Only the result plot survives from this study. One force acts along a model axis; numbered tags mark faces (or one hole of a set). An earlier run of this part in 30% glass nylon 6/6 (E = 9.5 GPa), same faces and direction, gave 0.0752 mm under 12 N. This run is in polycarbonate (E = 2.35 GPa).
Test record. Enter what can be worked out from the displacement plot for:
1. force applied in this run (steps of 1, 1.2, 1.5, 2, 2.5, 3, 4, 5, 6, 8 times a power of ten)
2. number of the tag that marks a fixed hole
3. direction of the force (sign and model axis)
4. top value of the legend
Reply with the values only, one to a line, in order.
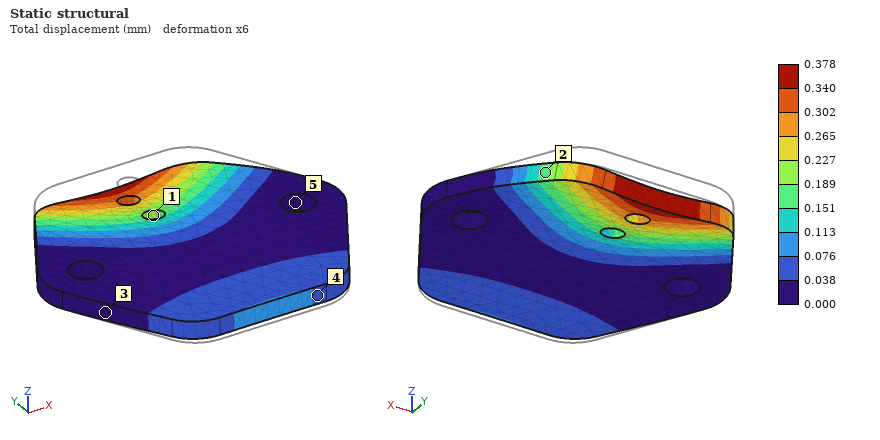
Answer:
15 N
5
-Z
0.378 mm
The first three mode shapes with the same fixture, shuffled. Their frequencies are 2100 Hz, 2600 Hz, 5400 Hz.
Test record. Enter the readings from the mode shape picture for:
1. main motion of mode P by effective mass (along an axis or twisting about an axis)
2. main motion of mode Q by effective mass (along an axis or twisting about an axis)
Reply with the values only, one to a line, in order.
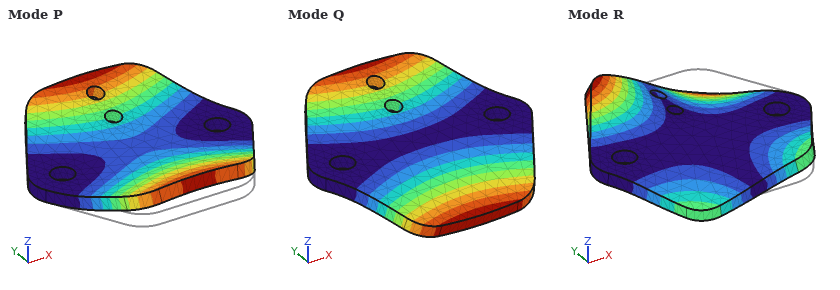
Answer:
along Z
twisting about X
